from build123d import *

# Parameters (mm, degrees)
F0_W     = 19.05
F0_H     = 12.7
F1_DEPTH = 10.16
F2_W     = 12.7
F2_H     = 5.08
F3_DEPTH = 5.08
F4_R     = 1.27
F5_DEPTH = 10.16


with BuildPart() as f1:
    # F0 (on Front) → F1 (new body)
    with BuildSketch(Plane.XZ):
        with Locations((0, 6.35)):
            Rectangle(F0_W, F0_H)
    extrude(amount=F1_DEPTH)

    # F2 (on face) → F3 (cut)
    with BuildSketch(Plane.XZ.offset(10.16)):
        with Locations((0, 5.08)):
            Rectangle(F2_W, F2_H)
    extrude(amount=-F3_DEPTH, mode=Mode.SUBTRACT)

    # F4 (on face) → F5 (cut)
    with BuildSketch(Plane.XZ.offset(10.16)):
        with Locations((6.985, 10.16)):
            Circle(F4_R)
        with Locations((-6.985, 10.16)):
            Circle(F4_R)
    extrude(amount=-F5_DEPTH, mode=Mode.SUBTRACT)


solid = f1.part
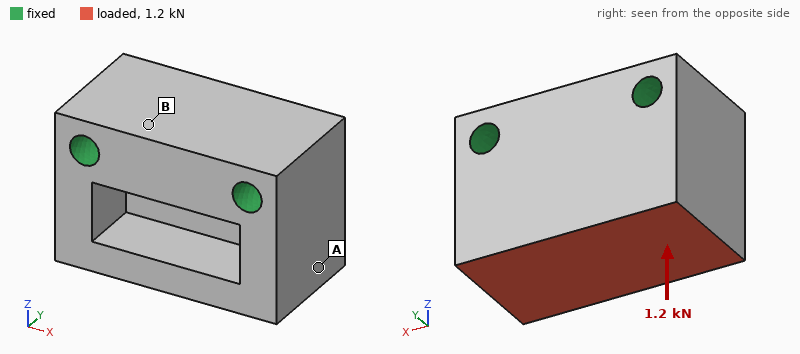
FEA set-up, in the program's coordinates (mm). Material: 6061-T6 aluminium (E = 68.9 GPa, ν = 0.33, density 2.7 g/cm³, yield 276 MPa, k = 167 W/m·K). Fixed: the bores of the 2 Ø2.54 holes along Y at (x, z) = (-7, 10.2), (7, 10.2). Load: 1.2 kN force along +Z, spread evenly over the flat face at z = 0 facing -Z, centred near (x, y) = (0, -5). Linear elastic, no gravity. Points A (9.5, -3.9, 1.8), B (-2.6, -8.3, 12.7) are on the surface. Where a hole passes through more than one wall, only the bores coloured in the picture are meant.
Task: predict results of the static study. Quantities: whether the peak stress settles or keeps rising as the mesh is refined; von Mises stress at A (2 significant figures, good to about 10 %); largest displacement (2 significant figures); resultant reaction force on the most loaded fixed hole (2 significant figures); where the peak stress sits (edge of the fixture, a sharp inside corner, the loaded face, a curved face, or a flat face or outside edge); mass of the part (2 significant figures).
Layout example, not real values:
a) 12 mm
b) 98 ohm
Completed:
a) keeps rising
b) 7.9 MPa
c) 10 µm
d) 610 N
e) a sharp inside corner
f) 5.5 g
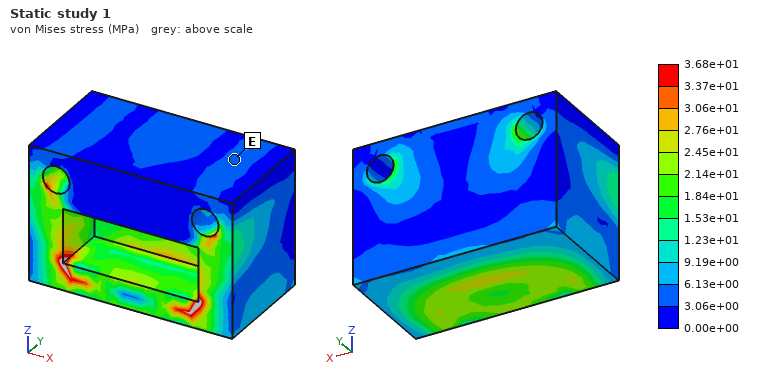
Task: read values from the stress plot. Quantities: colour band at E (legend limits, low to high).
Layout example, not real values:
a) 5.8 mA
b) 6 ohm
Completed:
a) 3.06e+00 to 6.13e+00 MPa
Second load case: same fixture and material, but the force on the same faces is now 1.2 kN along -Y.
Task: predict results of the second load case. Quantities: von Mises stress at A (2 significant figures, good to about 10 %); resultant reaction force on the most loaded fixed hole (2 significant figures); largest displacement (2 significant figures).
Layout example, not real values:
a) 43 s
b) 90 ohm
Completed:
a) 31 MPa
b) 600 N
c) 19 µm
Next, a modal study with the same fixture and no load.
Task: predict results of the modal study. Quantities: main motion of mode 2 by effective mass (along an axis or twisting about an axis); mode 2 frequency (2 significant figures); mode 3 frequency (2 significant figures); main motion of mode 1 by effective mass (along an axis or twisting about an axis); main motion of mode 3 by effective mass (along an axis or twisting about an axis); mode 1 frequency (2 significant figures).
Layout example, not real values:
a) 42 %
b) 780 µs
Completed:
a) along X
b) 47 kHz
c) 65 kHz
d) along Y
e) along X
f) 40 kHz
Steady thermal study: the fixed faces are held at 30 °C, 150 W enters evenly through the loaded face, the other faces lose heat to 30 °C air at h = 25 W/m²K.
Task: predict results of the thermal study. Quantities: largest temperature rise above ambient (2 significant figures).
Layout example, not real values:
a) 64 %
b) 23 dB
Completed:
a) 87 K
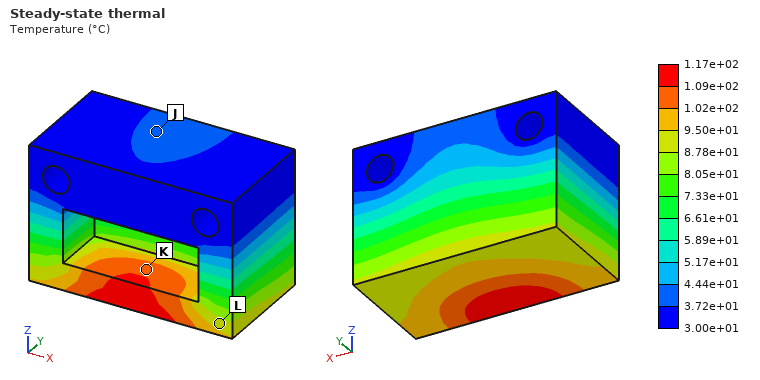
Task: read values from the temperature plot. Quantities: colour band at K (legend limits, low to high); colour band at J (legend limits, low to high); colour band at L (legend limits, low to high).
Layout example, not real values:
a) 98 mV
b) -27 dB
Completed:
a) 1.02e+02 to 1.09e+02 °C
b) 3.72e+01 to 4.44e+01 °C
c) 8.78e+01 to 9.50e+01 °C
